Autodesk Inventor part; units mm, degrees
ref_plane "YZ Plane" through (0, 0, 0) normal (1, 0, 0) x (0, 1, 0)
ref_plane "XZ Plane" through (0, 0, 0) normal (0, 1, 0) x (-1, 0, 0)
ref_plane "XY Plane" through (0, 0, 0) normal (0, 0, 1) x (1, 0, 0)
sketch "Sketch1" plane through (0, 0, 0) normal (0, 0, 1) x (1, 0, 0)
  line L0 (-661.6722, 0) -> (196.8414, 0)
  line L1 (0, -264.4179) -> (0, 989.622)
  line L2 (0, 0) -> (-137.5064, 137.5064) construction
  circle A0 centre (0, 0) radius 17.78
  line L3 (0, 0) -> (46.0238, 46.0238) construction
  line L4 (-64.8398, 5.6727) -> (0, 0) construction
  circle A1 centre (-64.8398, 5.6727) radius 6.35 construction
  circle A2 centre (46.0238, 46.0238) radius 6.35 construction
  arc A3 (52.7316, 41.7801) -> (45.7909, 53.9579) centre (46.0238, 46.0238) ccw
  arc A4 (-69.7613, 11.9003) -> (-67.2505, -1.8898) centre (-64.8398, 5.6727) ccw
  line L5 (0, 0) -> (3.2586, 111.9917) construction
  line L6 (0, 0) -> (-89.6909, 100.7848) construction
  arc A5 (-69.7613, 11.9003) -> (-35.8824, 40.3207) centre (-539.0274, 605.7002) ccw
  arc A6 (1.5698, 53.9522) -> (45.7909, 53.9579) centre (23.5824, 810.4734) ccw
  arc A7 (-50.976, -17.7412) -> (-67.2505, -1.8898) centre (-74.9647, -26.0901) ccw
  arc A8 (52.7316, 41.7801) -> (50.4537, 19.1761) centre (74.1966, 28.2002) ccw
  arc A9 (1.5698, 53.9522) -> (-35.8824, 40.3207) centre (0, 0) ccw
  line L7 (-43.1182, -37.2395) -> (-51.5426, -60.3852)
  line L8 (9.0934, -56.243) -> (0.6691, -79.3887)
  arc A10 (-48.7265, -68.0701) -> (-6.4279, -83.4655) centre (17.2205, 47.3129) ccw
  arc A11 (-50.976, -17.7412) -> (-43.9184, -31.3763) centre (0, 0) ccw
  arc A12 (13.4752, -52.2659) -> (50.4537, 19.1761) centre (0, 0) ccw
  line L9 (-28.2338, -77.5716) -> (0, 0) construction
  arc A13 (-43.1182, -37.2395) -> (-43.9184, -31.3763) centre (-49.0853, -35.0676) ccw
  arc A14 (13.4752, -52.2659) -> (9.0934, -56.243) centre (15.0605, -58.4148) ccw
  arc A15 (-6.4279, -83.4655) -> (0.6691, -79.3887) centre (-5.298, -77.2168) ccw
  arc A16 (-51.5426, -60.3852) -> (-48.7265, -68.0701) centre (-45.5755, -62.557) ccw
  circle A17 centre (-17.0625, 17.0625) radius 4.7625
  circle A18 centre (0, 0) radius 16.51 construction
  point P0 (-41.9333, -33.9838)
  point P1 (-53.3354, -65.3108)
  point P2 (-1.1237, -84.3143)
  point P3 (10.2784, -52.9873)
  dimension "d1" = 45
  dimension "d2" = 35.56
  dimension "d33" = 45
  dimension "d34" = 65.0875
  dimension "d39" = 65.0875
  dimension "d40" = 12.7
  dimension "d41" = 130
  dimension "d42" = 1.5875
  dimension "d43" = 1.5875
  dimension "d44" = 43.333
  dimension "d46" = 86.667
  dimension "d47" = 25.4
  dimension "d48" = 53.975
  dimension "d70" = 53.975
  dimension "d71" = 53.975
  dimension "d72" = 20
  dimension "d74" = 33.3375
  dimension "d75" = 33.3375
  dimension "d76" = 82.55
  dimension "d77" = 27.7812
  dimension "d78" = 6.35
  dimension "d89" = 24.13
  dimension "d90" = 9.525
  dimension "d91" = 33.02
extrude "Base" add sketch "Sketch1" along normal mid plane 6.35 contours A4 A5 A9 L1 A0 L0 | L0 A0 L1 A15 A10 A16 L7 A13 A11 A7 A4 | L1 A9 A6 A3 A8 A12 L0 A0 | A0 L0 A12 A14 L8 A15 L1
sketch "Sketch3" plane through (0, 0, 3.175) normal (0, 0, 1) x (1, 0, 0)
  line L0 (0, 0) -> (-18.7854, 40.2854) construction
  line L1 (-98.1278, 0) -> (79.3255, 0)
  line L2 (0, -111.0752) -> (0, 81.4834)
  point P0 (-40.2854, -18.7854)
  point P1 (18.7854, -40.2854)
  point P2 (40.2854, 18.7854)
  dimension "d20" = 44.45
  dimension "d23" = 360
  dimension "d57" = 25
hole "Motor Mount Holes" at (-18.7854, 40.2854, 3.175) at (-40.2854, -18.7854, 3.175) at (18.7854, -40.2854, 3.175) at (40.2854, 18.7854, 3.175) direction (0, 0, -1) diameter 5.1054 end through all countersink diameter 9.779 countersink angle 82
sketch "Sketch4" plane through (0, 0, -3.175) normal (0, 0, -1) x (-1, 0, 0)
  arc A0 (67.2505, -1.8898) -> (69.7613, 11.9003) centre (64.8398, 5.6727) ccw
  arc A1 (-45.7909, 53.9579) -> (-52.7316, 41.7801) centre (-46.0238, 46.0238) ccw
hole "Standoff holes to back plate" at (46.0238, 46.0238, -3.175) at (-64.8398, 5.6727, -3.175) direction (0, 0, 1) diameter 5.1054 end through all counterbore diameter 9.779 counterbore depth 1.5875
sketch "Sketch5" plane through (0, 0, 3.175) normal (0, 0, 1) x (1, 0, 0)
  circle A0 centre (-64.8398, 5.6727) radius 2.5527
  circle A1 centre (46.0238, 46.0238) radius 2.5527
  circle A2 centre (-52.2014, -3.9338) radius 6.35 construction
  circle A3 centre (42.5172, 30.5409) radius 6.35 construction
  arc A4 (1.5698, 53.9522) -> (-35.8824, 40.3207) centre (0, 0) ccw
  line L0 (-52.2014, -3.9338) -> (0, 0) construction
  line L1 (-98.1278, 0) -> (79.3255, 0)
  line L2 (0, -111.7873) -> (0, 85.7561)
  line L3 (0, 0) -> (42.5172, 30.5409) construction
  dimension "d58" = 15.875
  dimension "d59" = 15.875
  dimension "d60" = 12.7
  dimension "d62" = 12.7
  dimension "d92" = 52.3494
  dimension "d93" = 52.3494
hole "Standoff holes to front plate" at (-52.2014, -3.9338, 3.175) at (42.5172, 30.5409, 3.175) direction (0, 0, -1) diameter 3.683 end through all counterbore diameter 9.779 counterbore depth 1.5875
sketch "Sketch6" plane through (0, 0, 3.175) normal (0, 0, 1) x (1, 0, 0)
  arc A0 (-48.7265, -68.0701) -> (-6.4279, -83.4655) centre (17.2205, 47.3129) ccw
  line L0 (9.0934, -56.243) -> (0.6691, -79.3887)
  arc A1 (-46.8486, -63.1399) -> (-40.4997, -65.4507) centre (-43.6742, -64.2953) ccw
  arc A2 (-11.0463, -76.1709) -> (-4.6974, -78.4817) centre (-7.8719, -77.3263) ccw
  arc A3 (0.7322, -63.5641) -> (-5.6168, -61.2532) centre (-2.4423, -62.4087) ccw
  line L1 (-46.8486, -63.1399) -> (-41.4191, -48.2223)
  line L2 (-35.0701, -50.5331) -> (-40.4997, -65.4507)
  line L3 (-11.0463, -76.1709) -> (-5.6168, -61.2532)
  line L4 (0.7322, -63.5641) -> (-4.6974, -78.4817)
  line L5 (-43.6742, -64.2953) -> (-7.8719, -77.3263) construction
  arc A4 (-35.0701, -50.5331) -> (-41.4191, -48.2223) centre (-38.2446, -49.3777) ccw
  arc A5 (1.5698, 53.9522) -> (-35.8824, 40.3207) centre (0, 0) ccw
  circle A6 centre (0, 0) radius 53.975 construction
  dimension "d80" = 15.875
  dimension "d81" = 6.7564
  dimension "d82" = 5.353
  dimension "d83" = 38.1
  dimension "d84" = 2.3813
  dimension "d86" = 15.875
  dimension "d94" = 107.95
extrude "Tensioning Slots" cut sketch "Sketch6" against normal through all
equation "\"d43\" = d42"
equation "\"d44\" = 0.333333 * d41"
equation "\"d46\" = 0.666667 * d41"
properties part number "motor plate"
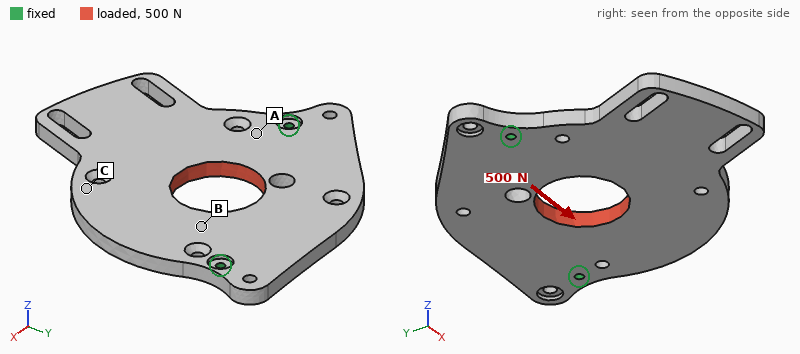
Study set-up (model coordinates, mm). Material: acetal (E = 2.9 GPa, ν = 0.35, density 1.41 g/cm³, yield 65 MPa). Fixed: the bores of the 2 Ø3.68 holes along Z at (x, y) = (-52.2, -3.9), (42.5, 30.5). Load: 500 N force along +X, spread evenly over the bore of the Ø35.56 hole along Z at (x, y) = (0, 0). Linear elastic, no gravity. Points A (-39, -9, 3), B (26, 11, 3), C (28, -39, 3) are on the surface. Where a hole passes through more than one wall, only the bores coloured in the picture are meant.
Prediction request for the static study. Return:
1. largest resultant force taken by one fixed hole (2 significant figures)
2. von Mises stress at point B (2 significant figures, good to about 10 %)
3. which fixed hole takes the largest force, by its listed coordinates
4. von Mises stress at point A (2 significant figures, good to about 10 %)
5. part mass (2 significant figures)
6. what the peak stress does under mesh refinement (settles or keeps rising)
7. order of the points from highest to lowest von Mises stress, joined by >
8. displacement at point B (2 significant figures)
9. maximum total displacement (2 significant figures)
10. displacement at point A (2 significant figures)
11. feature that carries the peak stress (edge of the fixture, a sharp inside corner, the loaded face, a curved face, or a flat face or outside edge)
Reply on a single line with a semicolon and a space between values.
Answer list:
280 N; 1.0 MPa; (-52.2, -3.9); 1.7 MPa; 91 g; keeps rising; A > B > C; 29 µm; 64 µm; 20 µm; edge of the fixture
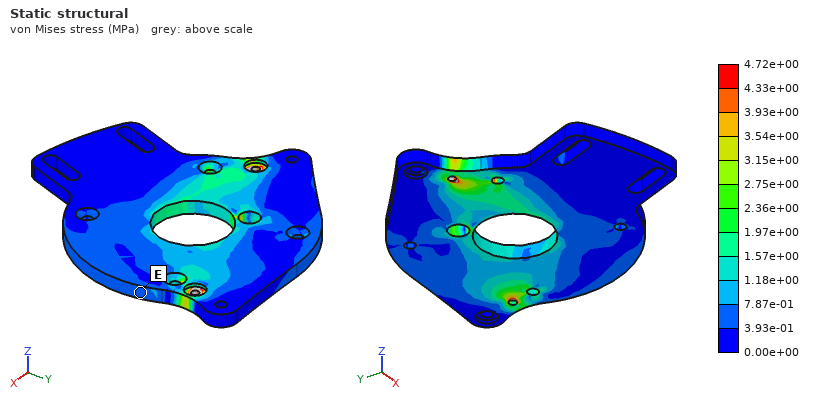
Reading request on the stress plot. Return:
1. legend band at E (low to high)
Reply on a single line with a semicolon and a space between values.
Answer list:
3.93e-01 to 7.87e-01 MPa
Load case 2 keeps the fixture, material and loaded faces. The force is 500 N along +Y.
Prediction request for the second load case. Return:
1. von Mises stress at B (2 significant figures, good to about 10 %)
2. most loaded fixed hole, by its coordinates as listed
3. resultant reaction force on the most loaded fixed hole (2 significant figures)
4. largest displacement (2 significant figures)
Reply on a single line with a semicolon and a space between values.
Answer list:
1.4 MPa; (42.5, 30.5); 270 N; 0.13 mm
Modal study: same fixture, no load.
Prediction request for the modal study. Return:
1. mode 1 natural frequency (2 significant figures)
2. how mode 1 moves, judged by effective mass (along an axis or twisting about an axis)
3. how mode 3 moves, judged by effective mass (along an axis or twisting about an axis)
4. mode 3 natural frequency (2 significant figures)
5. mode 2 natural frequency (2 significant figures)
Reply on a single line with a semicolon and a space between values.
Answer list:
160 Hz; along Z; along Z; 520 Hz; 450 Hz
